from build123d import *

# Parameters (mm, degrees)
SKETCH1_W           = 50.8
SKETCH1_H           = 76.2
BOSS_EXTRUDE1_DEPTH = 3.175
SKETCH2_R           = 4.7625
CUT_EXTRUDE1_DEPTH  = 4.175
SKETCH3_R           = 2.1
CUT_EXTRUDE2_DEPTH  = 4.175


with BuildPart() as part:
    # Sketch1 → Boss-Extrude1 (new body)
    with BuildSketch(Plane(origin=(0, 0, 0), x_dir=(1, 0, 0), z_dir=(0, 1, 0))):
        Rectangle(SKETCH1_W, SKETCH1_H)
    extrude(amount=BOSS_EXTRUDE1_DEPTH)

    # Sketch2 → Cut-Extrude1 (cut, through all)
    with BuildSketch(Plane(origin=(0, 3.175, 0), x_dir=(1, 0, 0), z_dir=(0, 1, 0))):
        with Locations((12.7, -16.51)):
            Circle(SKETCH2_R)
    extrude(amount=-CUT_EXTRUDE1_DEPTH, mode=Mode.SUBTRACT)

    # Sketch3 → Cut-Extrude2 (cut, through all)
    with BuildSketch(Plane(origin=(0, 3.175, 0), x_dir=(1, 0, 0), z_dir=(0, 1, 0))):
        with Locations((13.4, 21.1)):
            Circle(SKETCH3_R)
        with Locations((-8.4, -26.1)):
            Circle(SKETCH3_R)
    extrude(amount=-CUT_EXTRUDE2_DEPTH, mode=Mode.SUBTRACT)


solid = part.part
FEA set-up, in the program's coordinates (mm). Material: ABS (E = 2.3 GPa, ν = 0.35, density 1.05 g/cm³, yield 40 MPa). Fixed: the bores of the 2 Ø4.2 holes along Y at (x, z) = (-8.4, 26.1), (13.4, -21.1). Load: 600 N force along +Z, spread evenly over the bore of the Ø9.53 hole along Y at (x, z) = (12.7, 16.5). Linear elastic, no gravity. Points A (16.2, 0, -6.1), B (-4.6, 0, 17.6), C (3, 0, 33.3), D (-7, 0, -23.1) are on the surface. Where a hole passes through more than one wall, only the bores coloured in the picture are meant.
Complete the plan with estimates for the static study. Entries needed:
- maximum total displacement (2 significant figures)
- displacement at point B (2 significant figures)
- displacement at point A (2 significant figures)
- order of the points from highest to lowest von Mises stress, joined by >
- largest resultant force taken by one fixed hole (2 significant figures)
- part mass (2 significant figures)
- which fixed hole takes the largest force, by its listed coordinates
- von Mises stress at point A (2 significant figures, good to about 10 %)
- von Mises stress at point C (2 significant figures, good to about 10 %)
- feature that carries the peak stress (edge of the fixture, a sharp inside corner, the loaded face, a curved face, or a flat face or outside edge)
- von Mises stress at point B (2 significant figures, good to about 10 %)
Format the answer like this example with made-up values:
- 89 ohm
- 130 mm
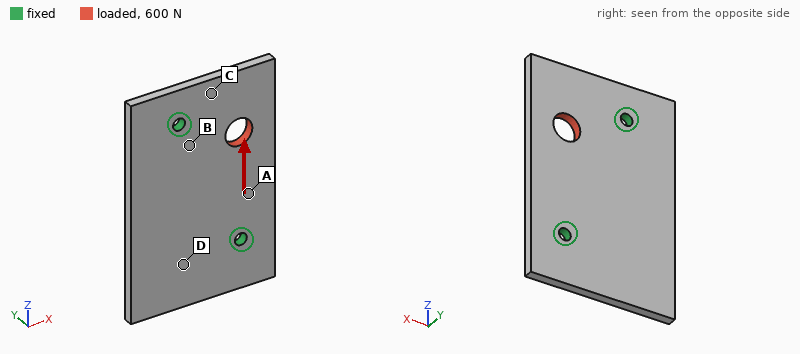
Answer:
- 0.13 mm
- 0.026 mm
- 0.043 mm
- A > B > C > D
- 350 N
- 13 g
- (13.4, -21.1)
- 6.0 MPa
- 2.5 MPa
- edge of the fixture
- 4.1 MPa
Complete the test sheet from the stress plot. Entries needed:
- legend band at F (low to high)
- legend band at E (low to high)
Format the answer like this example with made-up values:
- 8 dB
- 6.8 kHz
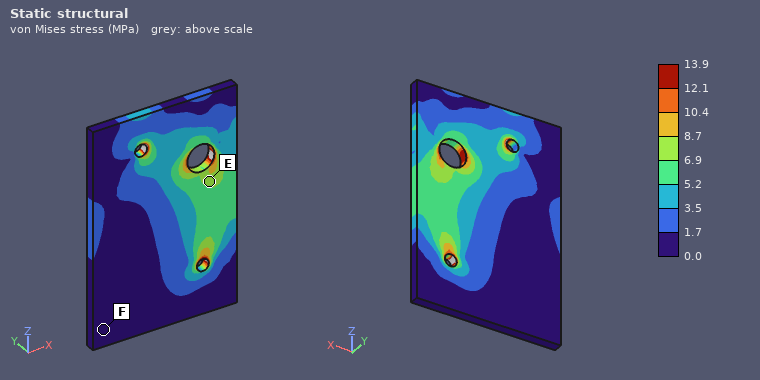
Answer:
- 0.0 to 1.7 MPa
- 6.9 to 8.7 MPa
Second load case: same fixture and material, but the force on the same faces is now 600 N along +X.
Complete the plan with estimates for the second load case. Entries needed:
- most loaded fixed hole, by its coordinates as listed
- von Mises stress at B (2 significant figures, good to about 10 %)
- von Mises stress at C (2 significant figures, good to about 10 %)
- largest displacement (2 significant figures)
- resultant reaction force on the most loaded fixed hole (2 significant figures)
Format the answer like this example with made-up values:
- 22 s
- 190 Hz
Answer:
- (-8.4, 26.1)
- 5.2 MPa
- 3.1 MPa
- 0.12 mm
- 470 N
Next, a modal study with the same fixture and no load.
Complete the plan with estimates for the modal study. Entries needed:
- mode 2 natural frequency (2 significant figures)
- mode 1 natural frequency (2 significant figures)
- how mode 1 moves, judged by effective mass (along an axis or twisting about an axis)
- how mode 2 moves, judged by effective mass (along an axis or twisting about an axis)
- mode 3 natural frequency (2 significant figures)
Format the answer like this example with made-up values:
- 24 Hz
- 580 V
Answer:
- 850 Hz
- 590 Hz
- along Y
- along Y
- 1300 Hz
